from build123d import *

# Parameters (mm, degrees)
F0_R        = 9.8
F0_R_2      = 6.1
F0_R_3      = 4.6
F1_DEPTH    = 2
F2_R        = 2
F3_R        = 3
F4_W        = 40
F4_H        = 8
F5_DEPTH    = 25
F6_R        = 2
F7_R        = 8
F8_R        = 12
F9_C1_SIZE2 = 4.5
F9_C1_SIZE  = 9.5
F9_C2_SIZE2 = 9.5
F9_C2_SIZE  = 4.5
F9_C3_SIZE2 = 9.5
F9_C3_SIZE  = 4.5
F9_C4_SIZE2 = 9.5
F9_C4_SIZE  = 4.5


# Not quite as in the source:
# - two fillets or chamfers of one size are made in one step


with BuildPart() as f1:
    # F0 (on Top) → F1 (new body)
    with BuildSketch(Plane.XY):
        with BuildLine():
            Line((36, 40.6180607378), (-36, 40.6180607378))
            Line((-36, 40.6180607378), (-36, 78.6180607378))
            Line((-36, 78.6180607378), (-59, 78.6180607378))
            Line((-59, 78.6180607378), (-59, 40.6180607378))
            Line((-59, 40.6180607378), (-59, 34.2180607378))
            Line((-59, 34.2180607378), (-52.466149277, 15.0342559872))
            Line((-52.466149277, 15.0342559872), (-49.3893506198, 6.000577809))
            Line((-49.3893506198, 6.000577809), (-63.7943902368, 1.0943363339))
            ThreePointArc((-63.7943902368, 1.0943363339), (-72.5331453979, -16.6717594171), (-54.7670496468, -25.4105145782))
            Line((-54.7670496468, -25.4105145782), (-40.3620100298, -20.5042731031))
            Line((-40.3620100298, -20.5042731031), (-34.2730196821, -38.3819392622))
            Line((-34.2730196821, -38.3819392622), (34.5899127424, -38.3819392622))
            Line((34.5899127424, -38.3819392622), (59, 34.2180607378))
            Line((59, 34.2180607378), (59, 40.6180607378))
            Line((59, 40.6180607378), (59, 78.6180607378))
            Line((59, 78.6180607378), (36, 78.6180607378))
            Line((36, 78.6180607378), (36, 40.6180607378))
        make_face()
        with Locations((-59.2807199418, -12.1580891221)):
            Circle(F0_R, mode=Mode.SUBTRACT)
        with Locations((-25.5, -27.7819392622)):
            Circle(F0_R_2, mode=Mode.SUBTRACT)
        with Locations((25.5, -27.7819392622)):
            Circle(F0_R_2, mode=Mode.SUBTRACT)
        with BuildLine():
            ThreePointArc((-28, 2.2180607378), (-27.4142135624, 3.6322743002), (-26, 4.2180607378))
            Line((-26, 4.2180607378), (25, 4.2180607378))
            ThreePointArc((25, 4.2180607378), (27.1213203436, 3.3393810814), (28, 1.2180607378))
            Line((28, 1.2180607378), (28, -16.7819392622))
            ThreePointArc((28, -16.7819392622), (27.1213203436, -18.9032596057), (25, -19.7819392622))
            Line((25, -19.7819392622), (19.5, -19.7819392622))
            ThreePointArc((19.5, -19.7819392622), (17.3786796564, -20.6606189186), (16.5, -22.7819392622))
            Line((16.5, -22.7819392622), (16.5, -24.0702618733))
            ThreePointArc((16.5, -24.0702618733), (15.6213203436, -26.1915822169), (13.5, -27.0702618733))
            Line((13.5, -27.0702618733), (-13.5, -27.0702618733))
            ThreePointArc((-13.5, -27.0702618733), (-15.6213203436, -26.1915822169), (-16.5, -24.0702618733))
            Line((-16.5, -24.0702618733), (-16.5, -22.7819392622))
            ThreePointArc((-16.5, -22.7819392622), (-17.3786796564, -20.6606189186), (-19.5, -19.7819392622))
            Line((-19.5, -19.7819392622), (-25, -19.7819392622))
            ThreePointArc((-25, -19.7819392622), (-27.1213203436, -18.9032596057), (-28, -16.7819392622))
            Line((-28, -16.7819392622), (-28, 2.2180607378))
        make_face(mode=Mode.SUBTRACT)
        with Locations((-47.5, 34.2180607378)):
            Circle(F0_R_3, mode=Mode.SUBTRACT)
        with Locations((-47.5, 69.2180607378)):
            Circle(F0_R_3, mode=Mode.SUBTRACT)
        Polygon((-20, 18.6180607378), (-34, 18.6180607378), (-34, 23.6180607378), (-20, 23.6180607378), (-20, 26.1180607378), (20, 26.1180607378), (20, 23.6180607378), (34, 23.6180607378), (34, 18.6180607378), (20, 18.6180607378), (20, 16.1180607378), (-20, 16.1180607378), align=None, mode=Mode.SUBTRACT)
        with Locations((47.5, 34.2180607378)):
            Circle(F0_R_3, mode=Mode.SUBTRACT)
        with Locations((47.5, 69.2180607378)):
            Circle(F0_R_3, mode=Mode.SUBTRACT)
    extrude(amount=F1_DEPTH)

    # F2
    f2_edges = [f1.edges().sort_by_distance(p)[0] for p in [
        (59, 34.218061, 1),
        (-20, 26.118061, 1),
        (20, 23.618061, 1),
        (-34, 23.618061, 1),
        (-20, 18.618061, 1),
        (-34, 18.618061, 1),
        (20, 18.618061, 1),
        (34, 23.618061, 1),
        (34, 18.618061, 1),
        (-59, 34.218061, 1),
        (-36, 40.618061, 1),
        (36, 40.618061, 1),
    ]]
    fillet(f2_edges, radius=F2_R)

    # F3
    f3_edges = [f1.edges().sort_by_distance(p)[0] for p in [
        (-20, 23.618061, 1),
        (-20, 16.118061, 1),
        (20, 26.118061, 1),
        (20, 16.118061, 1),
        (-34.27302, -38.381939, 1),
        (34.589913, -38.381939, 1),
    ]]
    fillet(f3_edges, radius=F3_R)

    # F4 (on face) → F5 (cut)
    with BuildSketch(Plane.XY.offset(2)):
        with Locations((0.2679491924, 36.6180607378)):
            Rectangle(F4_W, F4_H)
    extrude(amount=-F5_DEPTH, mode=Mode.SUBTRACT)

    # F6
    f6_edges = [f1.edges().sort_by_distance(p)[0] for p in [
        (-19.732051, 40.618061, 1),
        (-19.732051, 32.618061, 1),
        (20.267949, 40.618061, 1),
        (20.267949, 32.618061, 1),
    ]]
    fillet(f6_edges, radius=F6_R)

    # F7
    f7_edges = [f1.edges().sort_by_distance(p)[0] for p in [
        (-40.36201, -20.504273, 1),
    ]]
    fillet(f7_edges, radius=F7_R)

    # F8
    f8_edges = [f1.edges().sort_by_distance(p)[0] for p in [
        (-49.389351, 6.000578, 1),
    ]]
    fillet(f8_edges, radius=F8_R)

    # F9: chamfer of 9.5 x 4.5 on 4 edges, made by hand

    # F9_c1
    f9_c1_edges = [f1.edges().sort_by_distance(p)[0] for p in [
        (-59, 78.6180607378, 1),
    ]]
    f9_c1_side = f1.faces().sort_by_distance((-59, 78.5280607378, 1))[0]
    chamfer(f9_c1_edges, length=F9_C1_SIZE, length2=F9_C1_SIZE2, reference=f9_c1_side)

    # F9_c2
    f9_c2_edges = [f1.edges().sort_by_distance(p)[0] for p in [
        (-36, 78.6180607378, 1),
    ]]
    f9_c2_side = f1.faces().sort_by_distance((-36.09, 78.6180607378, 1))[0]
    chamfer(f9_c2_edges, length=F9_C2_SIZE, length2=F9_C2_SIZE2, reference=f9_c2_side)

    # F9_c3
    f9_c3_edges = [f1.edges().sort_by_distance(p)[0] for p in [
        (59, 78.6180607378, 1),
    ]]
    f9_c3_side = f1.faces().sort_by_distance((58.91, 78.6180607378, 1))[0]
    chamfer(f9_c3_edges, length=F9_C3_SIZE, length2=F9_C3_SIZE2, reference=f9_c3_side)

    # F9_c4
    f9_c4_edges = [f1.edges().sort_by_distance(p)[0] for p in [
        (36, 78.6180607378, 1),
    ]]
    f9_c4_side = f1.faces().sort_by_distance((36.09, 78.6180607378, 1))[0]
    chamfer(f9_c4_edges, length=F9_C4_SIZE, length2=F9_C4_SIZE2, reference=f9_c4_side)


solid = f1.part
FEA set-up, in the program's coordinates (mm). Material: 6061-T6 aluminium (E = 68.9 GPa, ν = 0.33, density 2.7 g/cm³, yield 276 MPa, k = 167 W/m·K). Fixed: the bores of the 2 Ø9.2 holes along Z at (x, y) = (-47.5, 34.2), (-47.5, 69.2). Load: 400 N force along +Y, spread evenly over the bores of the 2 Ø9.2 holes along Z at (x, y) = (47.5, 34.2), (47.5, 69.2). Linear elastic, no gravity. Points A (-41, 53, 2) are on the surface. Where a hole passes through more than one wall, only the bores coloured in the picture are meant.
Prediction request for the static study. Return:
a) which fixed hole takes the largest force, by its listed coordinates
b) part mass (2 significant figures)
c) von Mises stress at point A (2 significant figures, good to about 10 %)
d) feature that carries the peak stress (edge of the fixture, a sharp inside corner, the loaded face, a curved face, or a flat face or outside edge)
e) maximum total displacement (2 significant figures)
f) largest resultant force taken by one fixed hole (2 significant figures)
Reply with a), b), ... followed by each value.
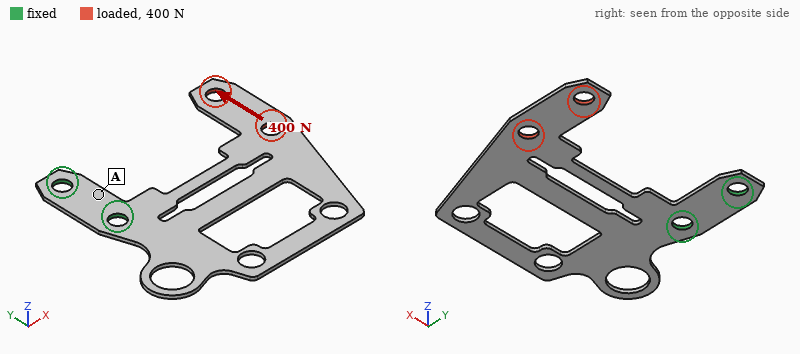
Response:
a) (-47.5, 69.2)
b) 36 g
c) 33 MPa
d) a curved face
e) 1.0 mm
f) 550 N
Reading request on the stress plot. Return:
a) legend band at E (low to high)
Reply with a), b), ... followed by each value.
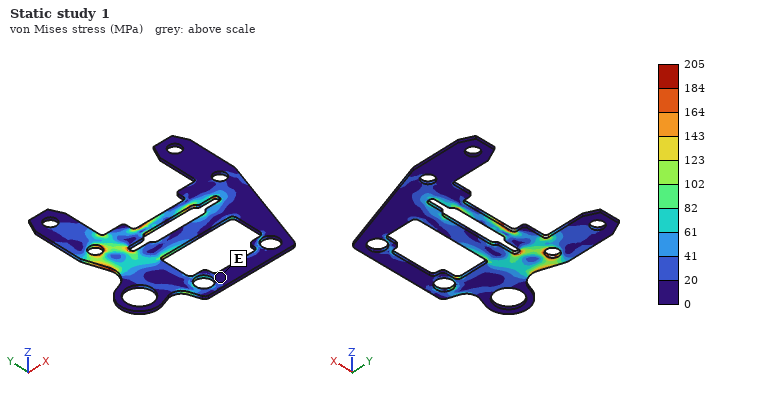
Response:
a) 0 to 20 MPa
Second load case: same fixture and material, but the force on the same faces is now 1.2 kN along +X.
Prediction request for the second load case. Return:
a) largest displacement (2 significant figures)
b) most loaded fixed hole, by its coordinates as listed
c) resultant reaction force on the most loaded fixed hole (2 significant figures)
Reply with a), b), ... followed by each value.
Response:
a) 1.2 mm
b) (-47.5, 34.2)
c) 940 N
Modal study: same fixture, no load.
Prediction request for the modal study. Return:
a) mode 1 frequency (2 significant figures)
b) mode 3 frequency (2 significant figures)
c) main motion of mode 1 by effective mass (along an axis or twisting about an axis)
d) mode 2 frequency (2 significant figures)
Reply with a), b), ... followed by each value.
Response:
a) 100 Hz
b) 450 Hz
c) along Z
d) 180 Hz
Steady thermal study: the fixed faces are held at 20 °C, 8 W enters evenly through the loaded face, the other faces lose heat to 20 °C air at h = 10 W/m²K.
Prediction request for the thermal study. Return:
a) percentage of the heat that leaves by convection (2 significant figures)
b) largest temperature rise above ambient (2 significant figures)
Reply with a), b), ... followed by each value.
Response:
a) 49 %
b) 76 K
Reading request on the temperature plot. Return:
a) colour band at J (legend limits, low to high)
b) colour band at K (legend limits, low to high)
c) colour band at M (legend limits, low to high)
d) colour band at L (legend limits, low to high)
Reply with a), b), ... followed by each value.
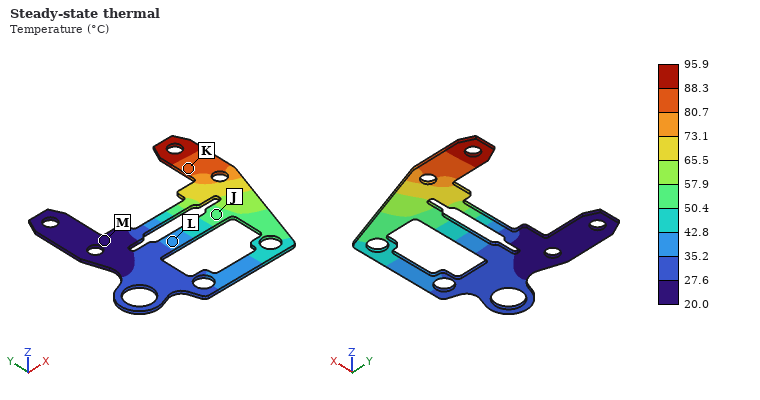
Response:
a) 50.4 to 57.9 °C
b) 80.7 to 88.3 °C
c) 20.0 to 27.6 °C
d) 35.2 to 42.8 °C
